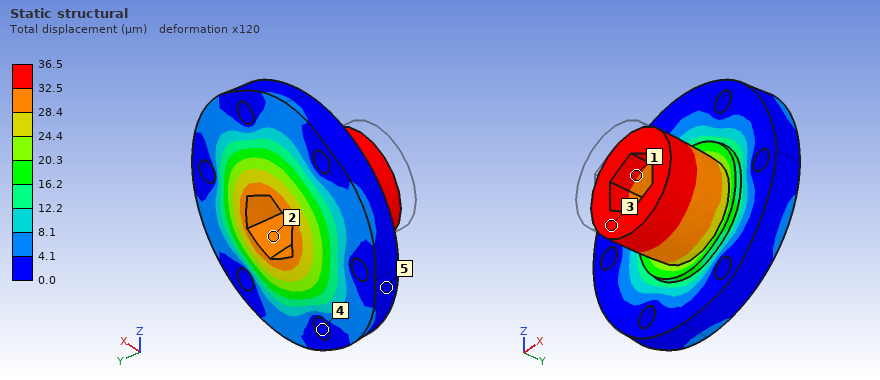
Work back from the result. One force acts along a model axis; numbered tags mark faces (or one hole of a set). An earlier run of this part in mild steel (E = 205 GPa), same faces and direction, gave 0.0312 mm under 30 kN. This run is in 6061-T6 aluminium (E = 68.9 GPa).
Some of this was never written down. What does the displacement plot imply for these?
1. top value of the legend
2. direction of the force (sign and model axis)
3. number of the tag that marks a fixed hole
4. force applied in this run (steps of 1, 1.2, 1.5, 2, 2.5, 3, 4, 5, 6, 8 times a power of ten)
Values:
36.5 µm
+Y
4
12 kN
